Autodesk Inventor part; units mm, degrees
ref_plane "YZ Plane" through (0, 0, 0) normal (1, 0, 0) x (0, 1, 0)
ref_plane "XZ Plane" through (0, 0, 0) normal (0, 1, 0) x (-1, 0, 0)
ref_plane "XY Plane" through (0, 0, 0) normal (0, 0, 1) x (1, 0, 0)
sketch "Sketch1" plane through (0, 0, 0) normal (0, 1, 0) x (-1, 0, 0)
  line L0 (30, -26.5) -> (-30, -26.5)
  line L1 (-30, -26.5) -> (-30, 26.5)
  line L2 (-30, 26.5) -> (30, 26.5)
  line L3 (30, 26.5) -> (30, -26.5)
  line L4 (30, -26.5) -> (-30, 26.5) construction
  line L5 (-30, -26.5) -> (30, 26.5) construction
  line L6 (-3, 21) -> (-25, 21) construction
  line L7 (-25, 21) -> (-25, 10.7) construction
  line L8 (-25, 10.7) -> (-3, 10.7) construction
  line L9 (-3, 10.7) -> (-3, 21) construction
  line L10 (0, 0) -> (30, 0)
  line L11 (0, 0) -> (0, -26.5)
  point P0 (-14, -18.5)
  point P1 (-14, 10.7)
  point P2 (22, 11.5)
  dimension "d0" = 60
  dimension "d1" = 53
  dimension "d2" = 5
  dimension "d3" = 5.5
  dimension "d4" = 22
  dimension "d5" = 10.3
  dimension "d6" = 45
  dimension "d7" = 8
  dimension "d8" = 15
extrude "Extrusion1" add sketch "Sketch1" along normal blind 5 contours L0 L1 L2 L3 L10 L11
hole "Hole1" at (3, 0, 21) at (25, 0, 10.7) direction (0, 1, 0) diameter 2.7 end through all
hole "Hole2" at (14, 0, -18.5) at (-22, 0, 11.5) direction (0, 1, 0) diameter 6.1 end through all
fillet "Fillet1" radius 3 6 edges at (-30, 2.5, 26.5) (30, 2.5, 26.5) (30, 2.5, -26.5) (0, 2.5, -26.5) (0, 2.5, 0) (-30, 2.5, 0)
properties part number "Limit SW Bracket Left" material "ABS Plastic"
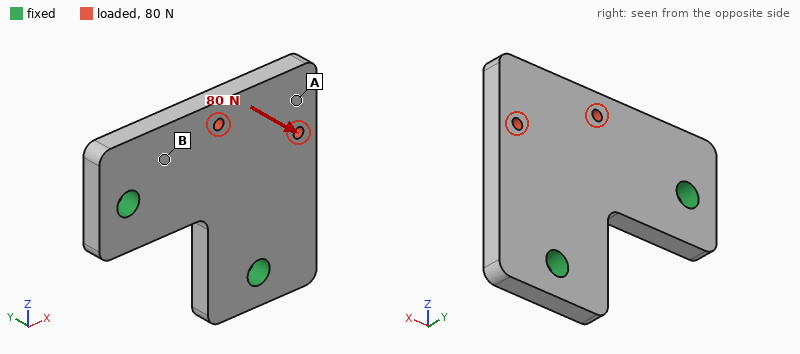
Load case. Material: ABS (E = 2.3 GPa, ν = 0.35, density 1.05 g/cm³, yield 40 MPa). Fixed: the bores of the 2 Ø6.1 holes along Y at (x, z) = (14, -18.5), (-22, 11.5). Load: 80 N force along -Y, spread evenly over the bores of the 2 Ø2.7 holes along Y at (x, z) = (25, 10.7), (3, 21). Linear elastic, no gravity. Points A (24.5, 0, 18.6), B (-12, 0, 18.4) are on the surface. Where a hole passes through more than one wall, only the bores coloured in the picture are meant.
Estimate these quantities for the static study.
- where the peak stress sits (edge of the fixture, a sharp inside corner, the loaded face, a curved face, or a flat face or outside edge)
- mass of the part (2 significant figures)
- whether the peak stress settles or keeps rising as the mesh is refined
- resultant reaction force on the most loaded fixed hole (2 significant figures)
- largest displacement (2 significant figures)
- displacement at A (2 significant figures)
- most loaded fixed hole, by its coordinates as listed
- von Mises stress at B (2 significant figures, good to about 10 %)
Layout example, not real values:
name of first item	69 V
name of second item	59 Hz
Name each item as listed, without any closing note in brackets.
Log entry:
where the peak stress sits	edge of the fixture
mass of the part	12 g
whether the peak stress settles or keeps rising as the mesh is refined	keeps rising
resultant reaction force on the most loaded fixed hole	42 N
largest displacement	0.90 mm
displacement at A	0.69 mm
most loaded fixed hole, by its coordinates as listed	(14, -18.5)
von Mises stress at B	5.3 MPa
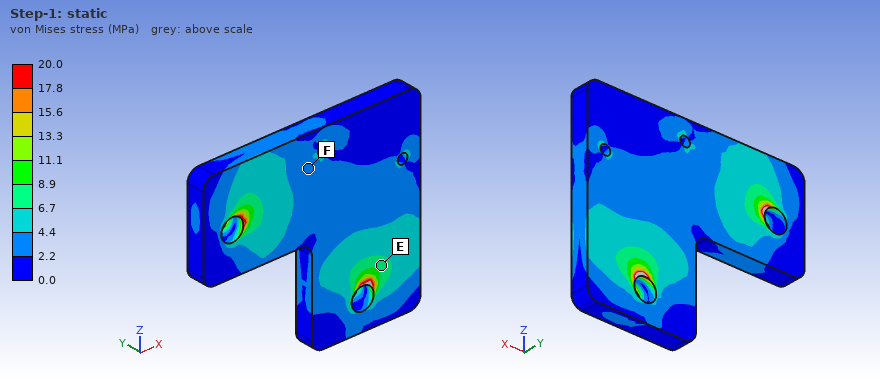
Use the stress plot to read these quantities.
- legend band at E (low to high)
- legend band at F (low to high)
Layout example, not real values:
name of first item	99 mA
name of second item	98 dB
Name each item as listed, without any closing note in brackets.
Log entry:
legend band at E	6.7 to 8.9 MPa
legend band at F	2.2 to 4.4 MPa
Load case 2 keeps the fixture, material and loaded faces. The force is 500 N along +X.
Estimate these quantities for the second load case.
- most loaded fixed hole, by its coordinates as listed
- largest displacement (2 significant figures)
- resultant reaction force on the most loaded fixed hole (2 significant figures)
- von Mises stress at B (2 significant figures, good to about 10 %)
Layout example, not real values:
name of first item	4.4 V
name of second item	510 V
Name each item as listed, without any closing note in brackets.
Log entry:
most loaded fixed hole, by its coordinates as listed	(-22, 11.5)
largest displacement	84 µm
resultant reaction force on the most loaded fixed hole	450 N
von Mises stress at B	4.7 MPa
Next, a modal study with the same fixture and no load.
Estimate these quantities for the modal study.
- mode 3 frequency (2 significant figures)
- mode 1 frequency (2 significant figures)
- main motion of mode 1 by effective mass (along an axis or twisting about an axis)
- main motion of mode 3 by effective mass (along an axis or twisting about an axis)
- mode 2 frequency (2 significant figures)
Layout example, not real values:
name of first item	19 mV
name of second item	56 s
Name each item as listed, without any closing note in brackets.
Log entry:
mode 3 frequency	3700 Hz
mode 1 frequency	940 Hz
main motion of mode 1 by effective mass	along Y
main motion of mode 3 by effective mass	along Y
mode 2 frequency	2800 Hz
